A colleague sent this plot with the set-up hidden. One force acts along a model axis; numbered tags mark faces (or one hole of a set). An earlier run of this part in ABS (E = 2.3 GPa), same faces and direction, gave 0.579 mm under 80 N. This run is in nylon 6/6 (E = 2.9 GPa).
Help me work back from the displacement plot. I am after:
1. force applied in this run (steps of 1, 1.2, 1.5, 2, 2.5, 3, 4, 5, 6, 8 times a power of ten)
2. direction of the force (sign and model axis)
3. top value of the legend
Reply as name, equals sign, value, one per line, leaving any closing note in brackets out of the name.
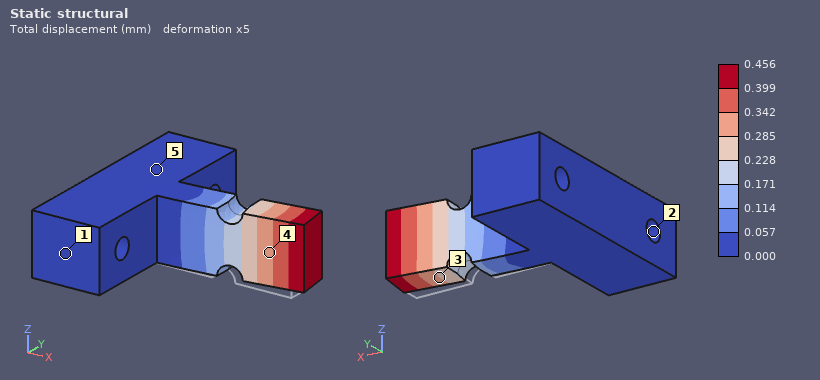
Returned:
force applied in this run = 80 N
direction of the force = +Y
top value of the legend = 0.456 mm
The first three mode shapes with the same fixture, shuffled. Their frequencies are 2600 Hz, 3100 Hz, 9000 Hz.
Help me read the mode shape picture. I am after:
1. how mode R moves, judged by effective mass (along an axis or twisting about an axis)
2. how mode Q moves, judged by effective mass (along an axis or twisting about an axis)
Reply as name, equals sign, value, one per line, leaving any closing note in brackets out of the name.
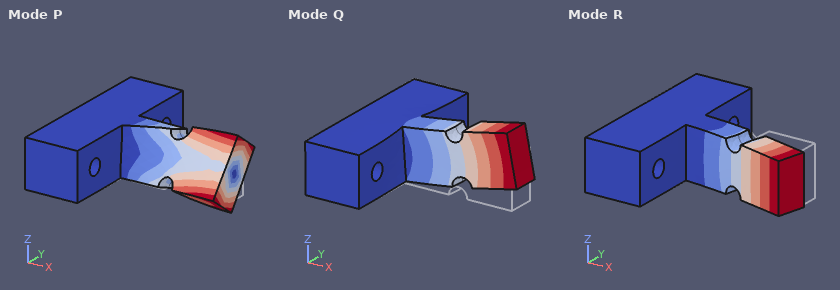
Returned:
how mode R moves, judged by effective mass = along Y
how mode Q moves, judged by effective mass = along Z
